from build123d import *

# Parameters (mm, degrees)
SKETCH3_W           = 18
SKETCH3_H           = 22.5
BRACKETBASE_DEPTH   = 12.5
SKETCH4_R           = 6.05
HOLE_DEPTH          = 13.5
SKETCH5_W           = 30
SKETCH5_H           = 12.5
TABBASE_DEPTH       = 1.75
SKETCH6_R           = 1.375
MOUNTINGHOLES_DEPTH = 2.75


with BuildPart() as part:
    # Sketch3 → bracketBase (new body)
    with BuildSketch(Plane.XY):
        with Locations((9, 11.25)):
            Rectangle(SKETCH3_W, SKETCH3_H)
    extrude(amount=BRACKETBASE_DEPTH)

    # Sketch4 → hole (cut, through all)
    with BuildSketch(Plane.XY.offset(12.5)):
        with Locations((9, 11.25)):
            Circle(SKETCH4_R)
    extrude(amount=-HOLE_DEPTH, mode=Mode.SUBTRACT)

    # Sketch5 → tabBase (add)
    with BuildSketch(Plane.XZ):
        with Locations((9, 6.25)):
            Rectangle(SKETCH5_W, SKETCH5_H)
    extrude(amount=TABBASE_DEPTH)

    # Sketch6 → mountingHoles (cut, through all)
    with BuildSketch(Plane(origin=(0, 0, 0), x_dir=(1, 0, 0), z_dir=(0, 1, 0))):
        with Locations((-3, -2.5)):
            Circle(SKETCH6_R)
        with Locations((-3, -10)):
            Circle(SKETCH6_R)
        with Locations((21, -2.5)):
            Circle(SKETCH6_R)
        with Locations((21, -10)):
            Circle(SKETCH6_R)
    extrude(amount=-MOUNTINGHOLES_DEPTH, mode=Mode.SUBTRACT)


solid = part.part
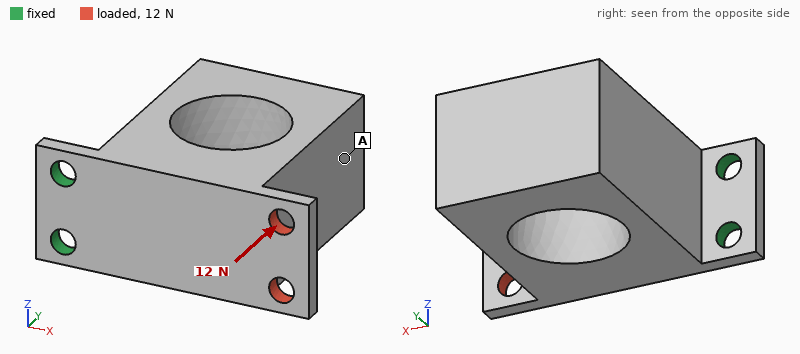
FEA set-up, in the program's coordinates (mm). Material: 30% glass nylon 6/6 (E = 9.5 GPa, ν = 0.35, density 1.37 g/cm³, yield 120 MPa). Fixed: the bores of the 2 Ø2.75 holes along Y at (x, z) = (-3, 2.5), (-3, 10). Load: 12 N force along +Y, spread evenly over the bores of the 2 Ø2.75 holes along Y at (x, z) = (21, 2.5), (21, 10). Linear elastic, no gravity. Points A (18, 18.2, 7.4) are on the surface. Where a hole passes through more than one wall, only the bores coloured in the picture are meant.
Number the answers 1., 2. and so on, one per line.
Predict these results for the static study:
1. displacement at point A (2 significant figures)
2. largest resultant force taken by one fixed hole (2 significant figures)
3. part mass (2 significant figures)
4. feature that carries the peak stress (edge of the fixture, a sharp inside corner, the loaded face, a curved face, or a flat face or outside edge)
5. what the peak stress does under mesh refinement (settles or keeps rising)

1. 0.38 mm
2. 6.1 N
3. 5.8 g
4. edge of the fixture
5. keeps rising
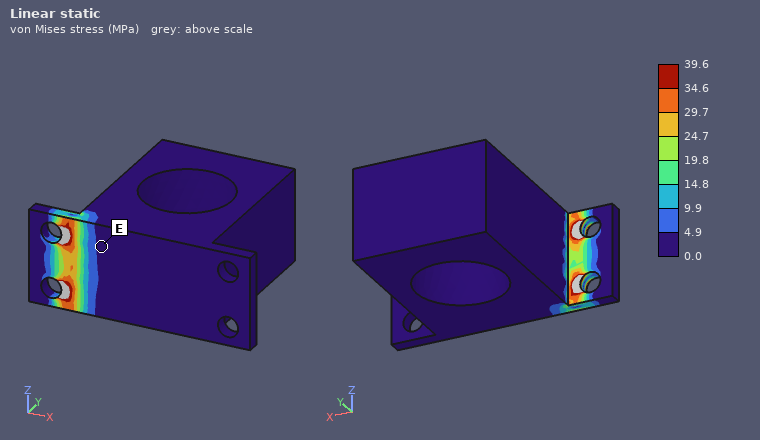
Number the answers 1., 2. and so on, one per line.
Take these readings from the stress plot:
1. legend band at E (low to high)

1. 0.0 to 4.9 MPa
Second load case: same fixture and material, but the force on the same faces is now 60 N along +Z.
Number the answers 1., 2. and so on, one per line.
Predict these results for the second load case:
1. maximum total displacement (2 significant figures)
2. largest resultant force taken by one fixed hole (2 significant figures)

1. 96 µm
2. 160 N
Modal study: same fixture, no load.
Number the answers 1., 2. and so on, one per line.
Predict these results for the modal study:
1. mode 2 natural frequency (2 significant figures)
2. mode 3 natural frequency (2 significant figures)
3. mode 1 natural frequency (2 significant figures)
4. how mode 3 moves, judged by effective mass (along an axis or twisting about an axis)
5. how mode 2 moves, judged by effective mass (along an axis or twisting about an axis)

1. 1800 Hz
2. 4400 Hz
3. 510 Hz
4. along Z
5. along Z
